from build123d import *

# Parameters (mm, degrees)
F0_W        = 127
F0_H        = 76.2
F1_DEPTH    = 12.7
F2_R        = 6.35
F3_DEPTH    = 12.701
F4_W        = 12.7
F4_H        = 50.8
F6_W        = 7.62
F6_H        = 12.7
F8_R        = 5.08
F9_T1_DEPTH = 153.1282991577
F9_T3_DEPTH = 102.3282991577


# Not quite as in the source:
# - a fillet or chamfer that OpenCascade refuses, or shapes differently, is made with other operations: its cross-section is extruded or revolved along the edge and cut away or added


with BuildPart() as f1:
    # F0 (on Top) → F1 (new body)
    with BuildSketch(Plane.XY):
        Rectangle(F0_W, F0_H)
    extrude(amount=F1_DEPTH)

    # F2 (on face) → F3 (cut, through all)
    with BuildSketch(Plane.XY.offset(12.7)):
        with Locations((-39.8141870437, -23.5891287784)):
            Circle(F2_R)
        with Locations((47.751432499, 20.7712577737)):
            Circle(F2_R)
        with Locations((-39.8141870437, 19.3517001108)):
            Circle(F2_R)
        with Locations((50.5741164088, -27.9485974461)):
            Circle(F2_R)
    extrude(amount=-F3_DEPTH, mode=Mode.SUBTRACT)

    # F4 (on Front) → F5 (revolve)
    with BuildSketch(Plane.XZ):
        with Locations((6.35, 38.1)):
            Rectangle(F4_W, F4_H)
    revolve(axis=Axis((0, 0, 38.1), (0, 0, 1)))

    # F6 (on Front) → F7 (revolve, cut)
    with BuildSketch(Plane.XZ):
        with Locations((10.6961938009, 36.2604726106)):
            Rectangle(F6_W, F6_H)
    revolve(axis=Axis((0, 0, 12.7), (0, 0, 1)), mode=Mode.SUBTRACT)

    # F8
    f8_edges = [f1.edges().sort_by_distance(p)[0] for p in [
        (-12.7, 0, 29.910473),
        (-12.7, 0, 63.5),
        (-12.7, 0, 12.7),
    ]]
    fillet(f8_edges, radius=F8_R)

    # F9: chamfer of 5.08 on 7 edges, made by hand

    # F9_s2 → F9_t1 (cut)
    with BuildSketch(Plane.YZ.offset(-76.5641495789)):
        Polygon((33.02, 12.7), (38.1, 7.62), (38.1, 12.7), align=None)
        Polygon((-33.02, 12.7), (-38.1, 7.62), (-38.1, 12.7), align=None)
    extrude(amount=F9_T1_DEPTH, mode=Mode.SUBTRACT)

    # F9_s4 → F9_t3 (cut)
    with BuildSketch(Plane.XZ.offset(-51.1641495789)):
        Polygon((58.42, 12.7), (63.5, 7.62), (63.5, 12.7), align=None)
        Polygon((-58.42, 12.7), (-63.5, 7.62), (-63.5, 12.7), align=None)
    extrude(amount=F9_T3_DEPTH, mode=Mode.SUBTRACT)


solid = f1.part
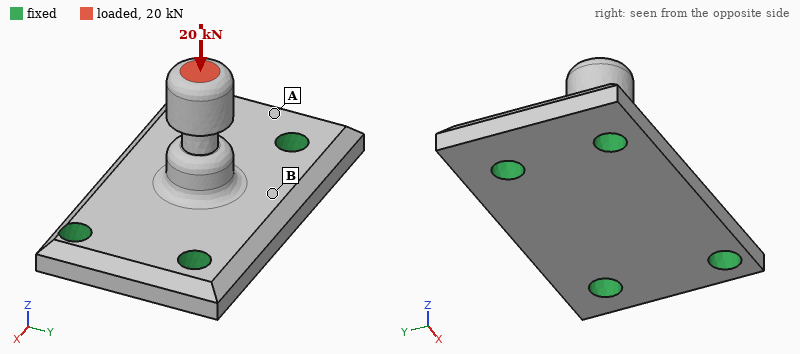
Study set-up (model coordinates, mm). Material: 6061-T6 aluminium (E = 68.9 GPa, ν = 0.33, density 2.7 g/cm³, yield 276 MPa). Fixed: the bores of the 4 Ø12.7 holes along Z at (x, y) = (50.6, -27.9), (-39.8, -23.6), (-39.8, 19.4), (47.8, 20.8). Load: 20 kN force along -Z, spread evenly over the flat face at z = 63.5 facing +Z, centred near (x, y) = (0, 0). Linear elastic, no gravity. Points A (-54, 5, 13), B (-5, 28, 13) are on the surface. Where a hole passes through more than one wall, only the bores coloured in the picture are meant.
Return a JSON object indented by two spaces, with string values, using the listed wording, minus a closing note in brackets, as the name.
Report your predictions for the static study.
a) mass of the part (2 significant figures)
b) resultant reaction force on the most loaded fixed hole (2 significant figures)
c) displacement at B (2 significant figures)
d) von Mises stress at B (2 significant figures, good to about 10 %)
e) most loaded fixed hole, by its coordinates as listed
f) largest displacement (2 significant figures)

{
  "mass of the part": "360 g",
  "resultant reaction force on the most loaded fixed hole": "6.2 kN",
  "displacement at B": "0.050 mm",
  "von Mises stress at B": "41 MPa",
  "most loaded fixed hole, by its coordinates as listed": "(-39.8, 19.4)",
  "largest displacement": "0.14 mm"
}
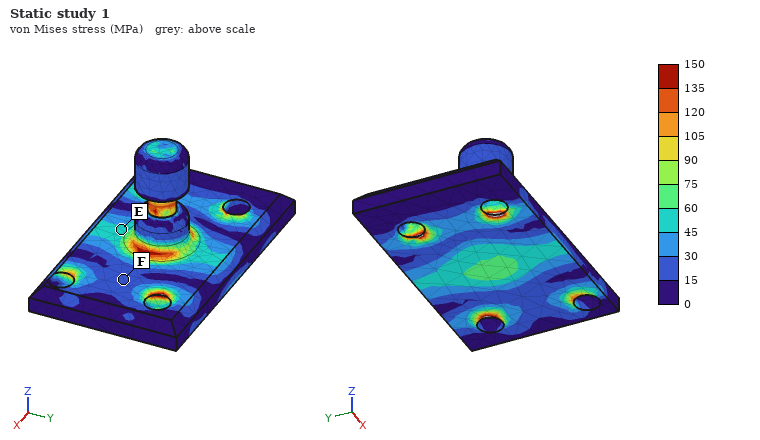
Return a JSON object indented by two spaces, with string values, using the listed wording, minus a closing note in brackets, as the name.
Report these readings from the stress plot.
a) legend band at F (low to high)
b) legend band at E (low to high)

{
  "legend band at F": "15 to 30 MPa",
  "legend band at E": "45 to 60 MPa"
}
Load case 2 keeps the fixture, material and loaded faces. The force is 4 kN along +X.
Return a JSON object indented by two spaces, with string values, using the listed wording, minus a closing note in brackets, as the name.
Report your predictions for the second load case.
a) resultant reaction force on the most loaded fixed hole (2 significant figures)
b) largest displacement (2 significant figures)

{
  "resultant reaction force on the most loaded fixed hole": "2.4 kN",
  "largest displacement": "0.64 mm"
}
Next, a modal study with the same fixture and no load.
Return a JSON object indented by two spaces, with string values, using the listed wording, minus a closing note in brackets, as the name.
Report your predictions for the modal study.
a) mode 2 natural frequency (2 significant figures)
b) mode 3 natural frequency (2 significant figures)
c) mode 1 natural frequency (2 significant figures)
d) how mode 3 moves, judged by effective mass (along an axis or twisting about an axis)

{
  "mode 2 natural frequency": "3300 Hz",
  "mode 3 natural frequency": "6900 Hz",
  "mode 1 natural frequency": "3200 Hz",
  "how mode 3 moves, judged by effective mass": "along Z"
}
